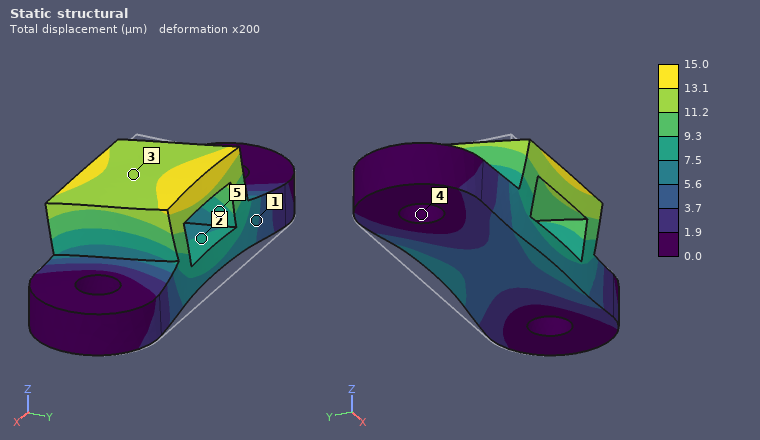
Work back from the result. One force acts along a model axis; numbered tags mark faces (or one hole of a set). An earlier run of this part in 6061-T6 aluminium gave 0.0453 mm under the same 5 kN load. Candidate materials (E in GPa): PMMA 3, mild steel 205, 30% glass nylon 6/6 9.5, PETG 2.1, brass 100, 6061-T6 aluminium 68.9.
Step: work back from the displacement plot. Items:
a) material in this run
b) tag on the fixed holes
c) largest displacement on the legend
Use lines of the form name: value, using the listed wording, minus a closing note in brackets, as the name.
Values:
material in this run: mild steel
tag on the fixed holes: 4
largest displacement on the legend: 15.0 µm
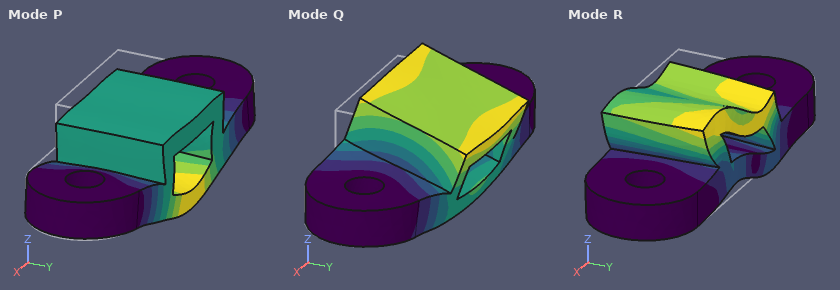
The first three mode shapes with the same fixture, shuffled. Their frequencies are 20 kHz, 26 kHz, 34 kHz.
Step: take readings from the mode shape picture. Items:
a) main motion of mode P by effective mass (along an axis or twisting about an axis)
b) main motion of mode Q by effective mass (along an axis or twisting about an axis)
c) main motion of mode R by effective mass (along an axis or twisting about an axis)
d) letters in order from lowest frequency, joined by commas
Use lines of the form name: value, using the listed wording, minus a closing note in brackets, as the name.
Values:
main motion of mode P by effective mass: along Z
main motion of mode Q by effective mass: along Y
main motion of mode R by effective mass: along X
letters in order from lowest frequency, joined by commas: Q, P, R
